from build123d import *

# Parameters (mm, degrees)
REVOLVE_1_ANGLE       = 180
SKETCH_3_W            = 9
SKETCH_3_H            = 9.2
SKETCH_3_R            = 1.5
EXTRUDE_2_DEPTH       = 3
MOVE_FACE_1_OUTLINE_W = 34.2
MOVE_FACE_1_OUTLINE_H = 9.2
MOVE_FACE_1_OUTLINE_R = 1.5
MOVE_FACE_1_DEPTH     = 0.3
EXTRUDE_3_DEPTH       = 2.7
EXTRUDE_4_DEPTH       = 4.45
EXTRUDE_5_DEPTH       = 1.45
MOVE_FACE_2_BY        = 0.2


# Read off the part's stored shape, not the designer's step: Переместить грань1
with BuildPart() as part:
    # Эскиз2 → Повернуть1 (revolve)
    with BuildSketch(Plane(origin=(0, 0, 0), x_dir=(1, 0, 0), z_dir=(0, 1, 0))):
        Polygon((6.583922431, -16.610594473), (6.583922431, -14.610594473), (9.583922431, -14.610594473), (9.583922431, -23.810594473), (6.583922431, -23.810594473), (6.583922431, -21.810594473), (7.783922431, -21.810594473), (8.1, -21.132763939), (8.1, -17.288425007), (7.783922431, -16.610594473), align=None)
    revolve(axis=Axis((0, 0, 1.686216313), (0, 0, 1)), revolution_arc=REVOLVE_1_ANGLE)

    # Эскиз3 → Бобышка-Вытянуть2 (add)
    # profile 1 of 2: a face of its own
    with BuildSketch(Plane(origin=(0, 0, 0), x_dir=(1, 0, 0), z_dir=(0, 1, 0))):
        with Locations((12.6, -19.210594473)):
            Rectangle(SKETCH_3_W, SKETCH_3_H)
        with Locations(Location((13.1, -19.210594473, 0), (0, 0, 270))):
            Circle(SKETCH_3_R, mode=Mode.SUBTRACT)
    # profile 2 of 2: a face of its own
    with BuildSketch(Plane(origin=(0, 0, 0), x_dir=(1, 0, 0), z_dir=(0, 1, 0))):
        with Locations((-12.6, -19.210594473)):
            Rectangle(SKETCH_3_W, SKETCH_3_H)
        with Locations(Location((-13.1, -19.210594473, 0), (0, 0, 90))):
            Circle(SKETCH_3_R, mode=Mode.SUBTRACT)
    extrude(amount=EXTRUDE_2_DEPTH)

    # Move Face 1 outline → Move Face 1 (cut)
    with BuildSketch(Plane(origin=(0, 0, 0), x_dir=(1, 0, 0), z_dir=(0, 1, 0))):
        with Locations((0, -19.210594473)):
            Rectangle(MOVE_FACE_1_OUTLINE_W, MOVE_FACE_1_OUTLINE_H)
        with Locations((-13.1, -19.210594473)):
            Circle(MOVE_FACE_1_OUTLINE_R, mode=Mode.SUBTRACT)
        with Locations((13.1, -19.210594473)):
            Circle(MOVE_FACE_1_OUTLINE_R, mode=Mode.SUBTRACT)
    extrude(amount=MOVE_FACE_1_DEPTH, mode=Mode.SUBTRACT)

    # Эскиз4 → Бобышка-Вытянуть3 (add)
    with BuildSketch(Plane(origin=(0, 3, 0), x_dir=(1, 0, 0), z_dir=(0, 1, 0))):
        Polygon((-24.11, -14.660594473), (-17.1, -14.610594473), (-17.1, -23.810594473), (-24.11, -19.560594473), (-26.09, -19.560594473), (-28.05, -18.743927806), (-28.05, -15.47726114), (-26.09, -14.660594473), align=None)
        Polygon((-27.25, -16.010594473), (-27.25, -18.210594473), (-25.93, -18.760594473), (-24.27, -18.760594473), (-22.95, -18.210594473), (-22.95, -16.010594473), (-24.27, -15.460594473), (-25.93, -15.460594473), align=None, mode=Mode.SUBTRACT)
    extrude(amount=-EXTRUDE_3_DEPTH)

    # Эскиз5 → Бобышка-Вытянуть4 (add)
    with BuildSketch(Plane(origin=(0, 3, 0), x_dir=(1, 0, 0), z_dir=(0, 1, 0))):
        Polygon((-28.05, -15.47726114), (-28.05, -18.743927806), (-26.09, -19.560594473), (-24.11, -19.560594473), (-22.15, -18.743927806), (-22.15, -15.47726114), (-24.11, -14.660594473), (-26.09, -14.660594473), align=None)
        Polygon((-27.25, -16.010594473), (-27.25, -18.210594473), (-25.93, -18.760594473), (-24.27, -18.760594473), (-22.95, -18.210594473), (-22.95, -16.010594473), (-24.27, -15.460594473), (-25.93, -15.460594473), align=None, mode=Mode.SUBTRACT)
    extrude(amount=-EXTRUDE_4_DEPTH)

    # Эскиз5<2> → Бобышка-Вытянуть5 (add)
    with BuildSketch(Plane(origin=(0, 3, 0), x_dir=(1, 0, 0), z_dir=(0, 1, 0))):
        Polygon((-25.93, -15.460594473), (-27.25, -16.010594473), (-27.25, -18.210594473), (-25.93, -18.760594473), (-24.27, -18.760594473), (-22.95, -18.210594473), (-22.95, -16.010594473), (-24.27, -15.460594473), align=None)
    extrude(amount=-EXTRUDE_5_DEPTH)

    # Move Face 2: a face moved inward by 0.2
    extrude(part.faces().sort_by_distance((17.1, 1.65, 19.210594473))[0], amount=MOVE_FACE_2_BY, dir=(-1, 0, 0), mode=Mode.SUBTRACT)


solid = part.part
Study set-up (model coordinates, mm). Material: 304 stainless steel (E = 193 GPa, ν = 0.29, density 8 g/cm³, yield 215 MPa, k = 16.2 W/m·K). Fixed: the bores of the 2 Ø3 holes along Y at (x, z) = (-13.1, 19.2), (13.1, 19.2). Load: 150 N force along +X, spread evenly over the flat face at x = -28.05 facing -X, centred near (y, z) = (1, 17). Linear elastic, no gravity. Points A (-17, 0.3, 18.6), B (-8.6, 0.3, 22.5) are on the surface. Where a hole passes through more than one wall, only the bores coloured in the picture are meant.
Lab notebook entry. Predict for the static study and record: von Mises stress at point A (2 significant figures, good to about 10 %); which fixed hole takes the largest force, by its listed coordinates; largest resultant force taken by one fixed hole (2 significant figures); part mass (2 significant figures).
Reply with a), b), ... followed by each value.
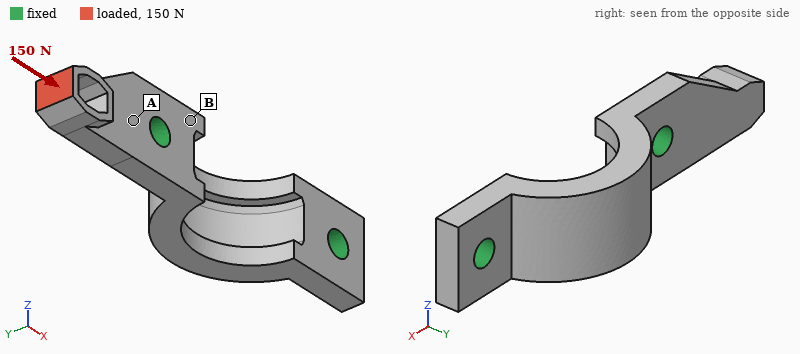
a) 22 MPa
b) (-13.1, 19.2)
c) 150 N
d) 8.3 g
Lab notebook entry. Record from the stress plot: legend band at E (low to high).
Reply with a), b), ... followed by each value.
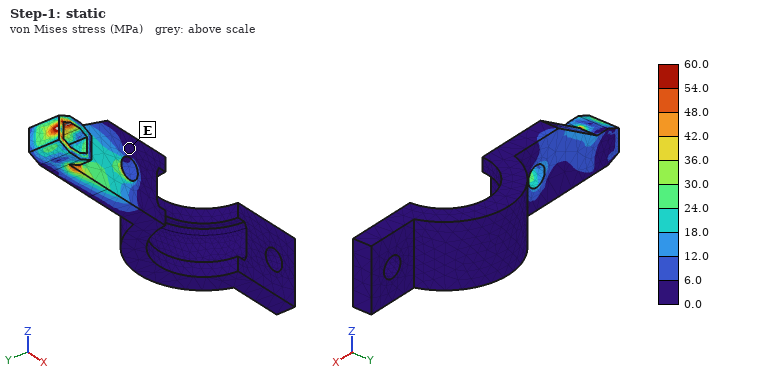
a) 0.0 to 6.0 MPa
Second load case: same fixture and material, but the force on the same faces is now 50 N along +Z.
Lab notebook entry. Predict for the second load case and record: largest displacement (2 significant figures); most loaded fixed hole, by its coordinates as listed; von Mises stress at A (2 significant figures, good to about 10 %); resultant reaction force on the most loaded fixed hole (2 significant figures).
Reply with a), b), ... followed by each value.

a) 6.5 µm
b) (-13.1, 19.2)
c) 8.9 MPa
d) 55 N
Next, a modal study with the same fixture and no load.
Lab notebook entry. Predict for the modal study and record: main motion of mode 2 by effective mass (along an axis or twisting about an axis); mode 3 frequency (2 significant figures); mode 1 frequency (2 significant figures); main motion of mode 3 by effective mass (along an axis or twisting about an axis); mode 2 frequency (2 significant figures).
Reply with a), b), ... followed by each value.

a) along Z
b) 25 kHz
c) 12 kHz
d) along Z
e) 18 kHz
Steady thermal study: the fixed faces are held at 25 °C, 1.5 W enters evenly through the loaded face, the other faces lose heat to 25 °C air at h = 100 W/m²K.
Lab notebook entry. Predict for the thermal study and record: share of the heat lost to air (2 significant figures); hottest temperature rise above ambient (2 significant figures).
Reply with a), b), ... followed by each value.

a) 51 %
b) 65 K
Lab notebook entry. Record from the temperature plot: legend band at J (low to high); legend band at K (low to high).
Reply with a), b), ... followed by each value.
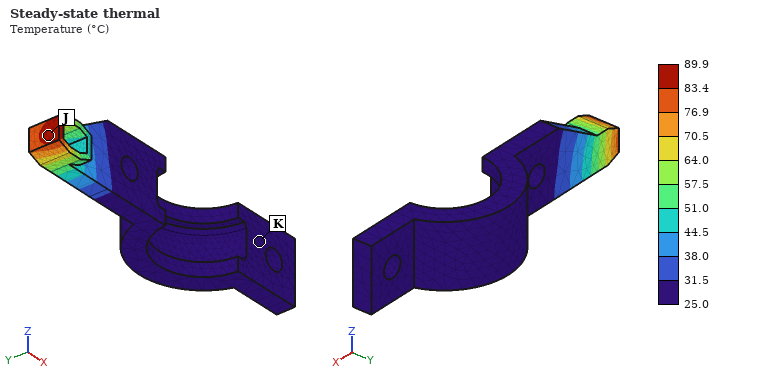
a) 83.4 to 89.9 °C
b) 25.0 to 31.5 °C
